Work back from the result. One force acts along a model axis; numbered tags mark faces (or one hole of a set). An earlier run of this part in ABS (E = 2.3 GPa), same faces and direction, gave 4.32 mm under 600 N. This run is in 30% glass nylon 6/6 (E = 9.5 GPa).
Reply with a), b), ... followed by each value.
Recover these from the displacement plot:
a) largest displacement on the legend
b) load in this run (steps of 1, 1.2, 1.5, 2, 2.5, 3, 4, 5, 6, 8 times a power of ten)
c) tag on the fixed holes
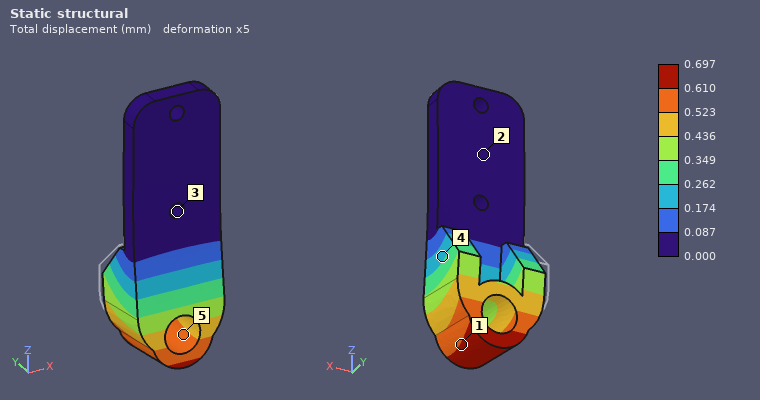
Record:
a) 0.697 mm
b) 400 N
c) 3
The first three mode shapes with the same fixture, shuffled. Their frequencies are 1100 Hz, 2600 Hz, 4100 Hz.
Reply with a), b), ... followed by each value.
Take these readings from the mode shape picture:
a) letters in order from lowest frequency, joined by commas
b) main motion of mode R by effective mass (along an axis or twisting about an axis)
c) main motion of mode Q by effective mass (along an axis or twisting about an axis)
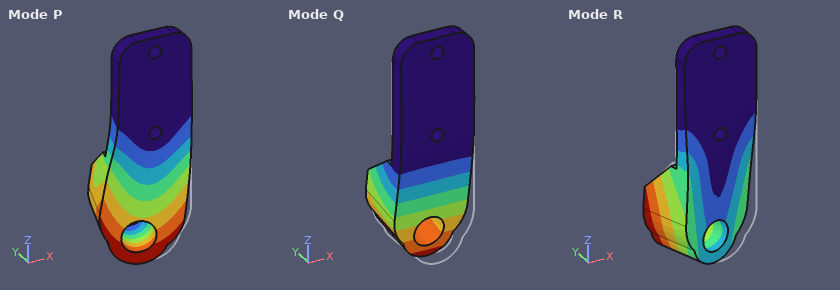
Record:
a) Q, R, P
b) along X
c) along Y
